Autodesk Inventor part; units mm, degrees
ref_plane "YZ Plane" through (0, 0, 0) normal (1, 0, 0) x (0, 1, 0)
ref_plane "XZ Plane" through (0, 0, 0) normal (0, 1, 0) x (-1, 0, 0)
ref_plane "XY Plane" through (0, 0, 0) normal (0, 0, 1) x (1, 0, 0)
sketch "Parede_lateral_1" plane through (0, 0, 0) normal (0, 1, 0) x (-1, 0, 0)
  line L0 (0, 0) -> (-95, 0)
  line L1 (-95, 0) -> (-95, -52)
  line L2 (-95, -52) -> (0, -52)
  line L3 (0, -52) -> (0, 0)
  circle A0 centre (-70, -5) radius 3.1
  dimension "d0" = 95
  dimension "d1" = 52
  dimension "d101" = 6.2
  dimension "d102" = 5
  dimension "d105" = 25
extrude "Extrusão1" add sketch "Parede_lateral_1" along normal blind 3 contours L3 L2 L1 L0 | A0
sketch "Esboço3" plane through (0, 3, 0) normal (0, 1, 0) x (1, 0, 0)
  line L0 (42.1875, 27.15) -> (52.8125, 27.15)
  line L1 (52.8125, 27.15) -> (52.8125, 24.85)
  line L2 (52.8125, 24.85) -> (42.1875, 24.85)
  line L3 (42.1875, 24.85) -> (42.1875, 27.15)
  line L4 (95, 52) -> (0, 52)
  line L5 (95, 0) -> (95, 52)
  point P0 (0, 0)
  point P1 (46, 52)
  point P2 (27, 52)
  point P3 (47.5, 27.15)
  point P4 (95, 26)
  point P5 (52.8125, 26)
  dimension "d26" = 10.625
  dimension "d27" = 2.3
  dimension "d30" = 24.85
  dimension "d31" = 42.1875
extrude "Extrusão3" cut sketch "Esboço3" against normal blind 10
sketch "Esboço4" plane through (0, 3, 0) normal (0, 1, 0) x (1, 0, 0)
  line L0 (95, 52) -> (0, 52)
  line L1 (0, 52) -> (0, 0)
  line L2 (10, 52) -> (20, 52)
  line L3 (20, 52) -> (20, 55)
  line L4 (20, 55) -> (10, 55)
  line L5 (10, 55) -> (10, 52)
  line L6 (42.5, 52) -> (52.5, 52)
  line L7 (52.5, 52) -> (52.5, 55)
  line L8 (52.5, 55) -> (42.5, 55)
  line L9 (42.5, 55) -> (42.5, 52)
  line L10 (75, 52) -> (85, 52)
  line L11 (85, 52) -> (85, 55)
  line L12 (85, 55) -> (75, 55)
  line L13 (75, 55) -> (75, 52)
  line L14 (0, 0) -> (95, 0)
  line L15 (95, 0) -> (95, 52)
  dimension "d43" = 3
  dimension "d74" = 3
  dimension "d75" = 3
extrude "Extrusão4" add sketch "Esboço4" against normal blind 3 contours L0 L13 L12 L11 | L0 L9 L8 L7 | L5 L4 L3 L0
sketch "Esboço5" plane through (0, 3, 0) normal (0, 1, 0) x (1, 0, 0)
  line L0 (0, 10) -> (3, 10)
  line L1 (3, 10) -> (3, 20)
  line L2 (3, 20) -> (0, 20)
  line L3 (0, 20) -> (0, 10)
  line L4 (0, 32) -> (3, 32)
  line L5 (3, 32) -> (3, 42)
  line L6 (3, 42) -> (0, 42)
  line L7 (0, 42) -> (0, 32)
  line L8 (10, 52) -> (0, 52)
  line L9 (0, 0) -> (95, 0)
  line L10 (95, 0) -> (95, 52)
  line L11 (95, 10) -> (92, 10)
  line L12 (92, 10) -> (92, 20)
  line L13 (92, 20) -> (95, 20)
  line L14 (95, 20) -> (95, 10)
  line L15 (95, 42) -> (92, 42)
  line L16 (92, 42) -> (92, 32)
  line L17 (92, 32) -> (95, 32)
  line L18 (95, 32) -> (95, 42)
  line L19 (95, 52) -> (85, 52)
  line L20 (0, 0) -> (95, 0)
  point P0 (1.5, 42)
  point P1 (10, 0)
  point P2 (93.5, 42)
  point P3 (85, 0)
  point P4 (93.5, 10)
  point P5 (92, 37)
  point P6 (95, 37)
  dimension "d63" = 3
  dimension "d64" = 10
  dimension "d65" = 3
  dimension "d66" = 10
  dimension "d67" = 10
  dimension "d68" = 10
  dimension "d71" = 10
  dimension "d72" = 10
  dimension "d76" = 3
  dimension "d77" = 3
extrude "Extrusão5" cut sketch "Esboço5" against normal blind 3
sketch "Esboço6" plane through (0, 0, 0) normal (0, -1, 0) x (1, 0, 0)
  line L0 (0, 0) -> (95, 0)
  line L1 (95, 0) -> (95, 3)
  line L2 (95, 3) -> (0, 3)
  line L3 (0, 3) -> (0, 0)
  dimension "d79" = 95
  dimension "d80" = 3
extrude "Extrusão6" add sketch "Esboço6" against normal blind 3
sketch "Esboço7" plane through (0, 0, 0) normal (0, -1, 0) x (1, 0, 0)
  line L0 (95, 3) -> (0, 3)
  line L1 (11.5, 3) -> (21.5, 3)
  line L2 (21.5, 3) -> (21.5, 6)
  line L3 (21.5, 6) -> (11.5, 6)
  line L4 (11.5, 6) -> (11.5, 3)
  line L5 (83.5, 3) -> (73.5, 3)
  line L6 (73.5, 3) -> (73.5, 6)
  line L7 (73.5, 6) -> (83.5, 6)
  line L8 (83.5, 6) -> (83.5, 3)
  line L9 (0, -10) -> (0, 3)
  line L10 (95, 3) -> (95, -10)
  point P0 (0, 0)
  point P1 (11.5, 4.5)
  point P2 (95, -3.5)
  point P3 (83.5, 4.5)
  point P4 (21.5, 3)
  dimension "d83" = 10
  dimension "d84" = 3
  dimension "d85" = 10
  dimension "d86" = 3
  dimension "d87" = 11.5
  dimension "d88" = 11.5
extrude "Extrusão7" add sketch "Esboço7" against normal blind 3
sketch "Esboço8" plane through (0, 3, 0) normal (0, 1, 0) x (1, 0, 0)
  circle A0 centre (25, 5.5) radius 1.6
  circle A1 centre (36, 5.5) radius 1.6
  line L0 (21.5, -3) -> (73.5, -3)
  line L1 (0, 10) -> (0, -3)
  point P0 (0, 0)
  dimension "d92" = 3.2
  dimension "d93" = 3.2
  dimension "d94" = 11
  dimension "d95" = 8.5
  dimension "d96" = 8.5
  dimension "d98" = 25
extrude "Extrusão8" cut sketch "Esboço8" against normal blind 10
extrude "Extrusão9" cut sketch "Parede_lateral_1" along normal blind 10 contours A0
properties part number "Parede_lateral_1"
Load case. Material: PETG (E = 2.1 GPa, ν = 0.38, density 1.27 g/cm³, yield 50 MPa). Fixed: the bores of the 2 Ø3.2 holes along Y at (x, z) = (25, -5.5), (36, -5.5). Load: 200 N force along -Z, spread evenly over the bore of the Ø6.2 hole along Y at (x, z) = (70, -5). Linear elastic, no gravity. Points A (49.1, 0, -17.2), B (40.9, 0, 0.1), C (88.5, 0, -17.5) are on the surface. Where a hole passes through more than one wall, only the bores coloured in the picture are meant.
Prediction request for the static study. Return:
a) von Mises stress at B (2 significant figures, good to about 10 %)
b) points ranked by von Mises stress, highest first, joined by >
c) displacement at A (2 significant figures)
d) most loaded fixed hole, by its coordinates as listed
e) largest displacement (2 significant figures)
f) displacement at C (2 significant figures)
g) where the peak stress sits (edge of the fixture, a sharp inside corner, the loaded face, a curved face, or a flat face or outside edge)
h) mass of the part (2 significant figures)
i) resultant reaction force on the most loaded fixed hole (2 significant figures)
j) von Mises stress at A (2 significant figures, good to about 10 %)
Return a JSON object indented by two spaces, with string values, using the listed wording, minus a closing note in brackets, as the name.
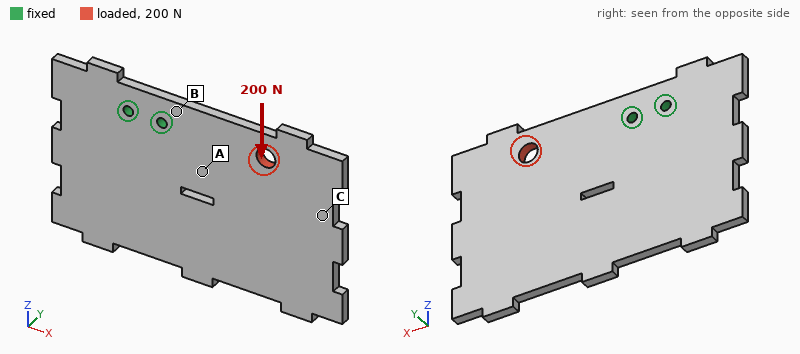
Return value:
{
  "von Mises stress at B": "9.3 MPa",
  "points ranked by von Mises stress, highest first, joined by >": "B > A > C",
  "displacement at A": "0.31 mm",
  "most loaded fixed hole, by its coordinates as listed": "(36, -5.5)",
  "largest displacement": "1.2 mm",
  "displacement at C": "0.93 mm",
  "where the peak stress sits": "edge of the fixture",
  "mass of the part": "20 g",
  "resultant reaction force on the most loaded fixed hole": "680 N",
  "von Mises stress at A": "4.8 MPa"
}
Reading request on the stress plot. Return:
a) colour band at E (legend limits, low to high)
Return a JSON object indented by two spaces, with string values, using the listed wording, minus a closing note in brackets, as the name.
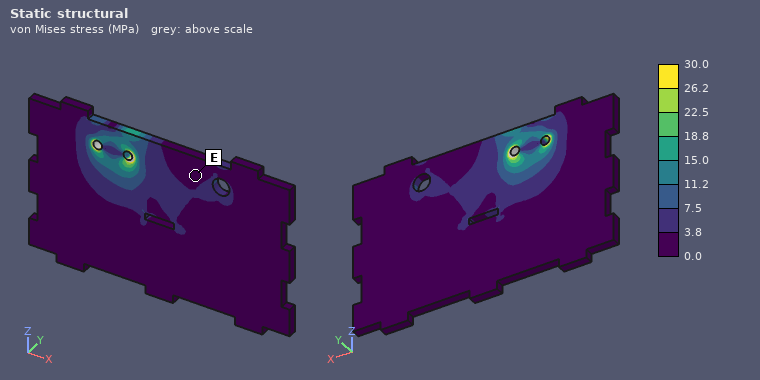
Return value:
{
  "colour band at E": "0.0 to 3.8 MPa"
}
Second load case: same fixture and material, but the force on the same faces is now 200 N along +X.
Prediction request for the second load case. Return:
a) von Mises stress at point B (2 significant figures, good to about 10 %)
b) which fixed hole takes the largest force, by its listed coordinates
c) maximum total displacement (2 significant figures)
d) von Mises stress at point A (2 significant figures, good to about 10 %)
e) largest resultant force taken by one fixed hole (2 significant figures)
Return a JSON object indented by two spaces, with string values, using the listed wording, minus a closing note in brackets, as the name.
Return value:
{
  "von Mises stress at point B": "3.2 MPa",
  "which fixed hole takes the largest force, by its listed coordinates": "(36, -5.5)",
  "maximum total displacement": "0.10 mm",
  "von Mises stress at point A": "1.6 MPa",
  "largest resultant force taken by one fixed hole": "150 N"
}
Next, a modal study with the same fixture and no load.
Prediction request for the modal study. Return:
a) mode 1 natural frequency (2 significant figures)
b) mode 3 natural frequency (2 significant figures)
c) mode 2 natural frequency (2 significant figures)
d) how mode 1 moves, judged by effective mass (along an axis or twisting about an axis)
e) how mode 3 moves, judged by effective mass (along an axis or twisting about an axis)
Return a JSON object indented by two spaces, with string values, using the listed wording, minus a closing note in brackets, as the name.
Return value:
{
  "mode 1 natural frequency": "130 Hz",
  "mode 3 natural frequency": "400 Hz",
  "mode 2 natural frequency": "230 Hz",
  "how mode 1 moves, judged by effective mass": "along Y",
  "how mode 3 moves, judged by effective mass": "along Y"
}
